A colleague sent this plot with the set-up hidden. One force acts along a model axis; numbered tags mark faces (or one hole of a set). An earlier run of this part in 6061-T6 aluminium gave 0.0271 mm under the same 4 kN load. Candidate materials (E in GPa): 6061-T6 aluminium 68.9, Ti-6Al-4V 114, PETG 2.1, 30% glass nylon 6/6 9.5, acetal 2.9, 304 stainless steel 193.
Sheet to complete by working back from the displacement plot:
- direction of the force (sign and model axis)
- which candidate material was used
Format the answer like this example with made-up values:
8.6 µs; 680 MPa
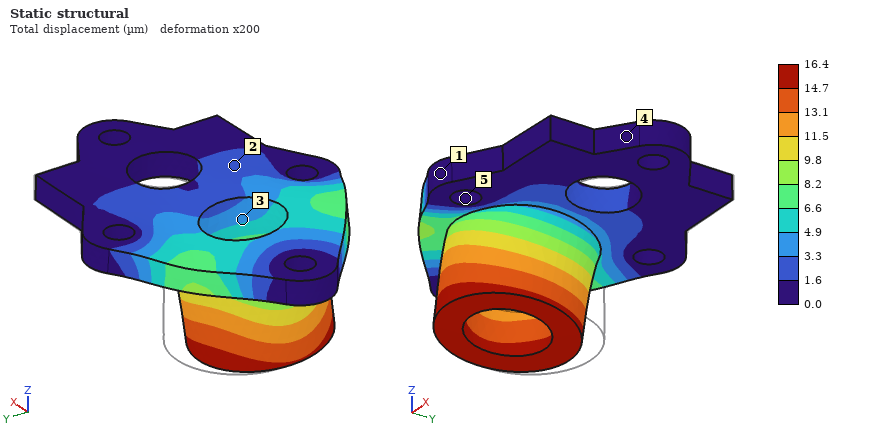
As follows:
-Y; Ti-6Al-4V
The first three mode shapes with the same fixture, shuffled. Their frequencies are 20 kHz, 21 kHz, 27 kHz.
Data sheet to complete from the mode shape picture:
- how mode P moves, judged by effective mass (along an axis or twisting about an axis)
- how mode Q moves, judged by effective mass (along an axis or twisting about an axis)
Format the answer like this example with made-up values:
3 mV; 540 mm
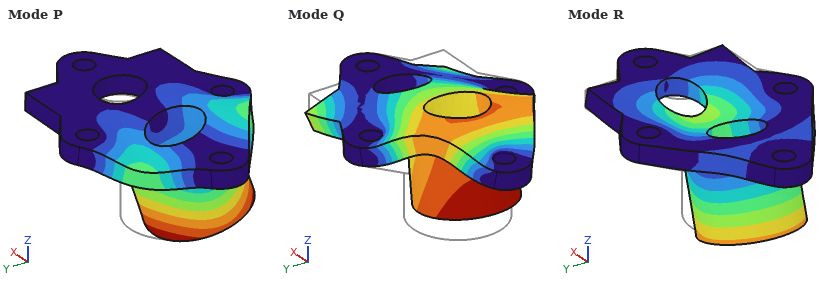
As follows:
along Y; along Z
